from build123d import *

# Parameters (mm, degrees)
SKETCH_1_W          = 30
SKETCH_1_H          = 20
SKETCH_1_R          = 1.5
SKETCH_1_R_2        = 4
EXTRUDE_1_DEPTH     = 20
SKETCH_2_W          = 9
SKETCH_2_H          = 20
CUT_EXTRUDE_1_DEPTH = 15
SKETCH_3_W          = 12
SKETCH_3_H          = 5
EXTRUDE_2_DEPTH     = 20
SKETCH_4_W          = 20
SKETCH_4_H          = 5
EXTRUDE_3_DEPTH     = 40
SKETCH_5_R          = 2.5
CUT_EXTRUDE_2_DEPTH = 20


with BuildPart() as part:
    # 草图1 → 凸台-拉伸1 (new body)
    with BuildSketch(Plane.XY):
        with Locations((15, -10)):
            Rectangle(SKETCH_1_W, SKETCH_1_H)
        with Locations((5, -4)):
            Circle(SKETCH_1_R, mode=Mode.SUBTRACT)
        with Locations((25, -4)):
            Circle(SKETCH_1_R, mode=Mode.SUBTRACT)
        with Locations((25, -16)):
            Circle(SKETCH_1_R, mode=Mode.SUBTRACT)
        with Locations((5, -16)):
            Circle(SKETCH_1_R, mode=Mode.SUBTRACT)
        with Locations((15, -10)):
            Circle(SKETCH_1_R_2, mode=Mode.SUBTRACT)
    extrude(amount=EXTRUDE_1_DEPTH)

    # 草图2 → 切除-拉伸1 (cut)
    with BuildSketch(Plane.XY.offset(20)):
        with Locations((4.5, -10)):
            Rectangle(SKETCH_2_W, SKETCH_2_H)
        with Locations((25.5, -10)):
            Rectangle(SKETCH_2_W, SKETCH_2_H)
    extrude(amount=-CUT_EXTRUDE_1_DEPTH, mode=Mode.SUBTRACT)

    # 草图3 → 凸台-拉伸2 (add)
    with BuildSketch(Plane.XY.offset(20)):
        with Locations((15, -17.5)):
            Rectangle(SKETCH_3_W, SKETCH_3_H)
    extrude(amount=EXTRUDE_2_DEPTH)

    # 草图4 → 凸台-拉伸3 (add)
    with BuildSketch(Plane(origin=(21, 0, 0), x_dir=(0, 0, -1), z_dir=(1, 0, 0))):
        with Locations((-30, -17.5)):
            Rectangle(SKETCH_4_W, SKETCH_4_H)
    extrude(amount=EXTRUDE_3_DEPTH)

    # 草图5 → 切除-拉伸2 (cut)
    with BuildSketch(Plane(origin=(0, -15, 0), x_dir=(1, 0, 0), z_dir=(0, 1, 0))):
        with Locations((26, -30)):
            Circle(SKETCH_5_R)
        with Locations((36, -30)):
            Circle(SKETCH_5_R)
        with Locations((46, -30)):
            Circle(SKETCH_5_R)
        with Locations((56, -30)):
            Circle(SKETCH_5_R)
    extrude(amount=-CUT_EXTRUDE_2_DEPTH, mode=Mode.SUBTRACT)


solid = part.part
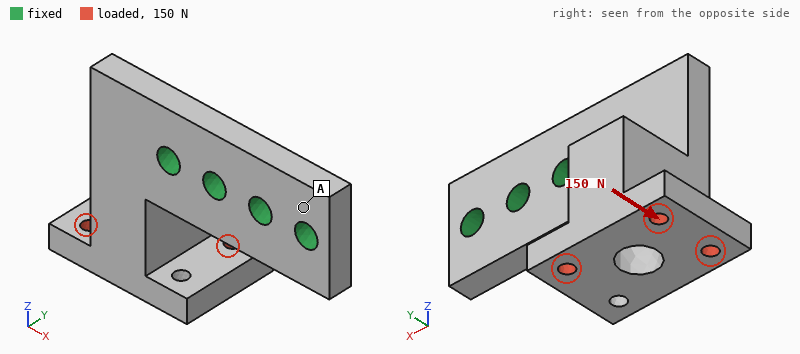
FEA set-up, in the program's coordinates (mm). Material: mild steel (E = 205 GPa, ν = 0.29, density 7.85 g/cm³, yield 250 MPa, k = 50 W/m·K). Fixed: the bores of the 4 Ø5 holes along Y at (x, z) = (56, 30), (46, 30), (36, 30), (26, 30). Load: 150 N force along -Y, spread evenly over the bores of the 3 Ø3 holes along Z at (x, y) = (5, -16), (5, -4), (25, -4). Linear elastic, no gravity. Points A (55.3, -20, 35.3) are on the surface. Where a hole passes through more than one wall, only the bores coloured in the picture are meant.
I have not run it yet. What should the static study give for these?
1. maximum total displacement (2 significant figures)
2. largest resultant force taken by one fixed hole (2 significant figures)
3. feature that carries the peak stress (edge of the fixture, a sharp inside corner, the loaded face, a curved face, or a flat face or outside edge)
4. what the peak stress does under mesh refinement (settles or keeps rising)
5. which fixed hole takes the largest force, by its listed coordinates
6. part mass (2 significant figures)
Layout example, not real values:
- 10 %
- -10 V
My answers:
- 57 µm
- 200 N
- edge of the fixture
- keeps rising
- (26, 30)
- 81 g
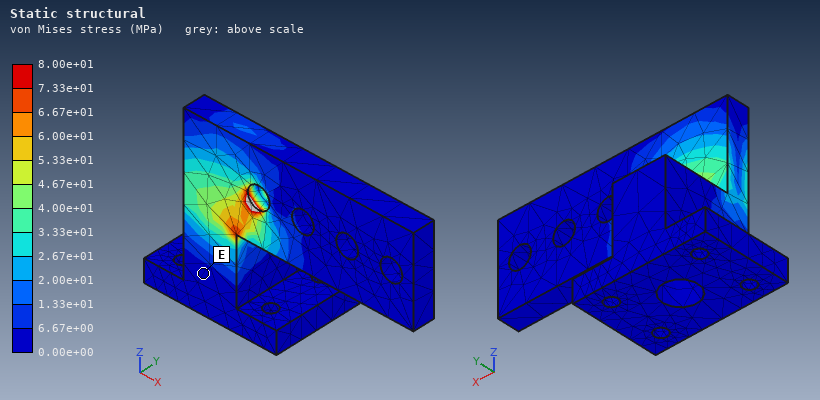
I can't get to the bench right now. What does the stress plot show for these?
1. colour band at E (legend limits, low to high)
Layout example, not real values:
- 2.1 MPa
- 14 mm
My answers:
- 0.00e+00 to 6.67e+00 MPa
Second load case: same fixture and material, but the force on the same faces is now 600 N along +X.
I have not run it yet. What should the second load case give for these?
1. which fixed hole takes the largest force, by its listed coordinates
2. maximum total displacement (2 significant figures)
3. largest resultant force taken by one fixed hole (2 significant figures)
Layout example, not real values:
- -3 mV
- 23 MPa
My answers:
- (26, 30)
- 83 µm
- 810 N
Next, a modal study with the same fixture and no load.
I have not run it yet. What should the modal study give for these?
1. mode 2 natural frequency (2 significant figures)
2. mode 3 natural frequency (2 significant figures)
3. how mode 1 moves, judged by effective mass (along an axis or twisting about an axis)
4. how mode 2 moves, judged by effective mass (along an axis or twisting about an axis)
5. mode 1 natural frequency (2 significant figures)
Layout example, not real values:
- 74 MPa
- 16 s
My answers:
- 3000 Hz
- 5400 Hz
- along Y
- along X
- 1700 Hz
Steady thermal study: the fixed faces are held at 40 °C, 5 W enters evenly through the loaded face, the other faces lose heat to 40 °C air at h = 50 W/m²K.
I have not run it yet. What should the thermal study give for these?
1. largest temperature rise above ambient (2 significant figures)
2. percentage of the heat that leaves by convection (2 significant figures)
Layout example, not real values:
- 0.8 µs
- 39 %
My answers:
- 23 K
- 53 %
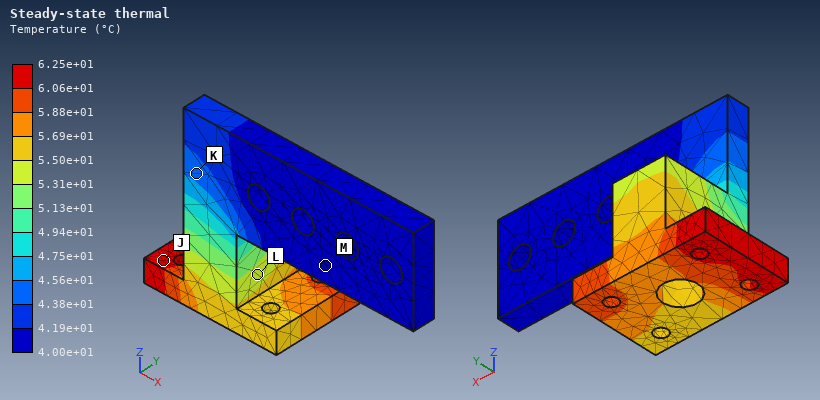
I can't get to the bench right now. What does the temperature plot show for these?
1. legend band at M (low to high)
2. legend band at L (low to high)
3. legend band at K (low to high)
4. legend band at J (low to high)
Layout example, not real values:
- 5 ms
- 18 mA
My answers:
- 4.00e+01 to 4.19e+01 °C
- 5.31e+01 to 5.50e+01 °C
- 4.38e+01 to 4.56e+01 °C
- 6.06e+01 to 6.25e+01 °C
